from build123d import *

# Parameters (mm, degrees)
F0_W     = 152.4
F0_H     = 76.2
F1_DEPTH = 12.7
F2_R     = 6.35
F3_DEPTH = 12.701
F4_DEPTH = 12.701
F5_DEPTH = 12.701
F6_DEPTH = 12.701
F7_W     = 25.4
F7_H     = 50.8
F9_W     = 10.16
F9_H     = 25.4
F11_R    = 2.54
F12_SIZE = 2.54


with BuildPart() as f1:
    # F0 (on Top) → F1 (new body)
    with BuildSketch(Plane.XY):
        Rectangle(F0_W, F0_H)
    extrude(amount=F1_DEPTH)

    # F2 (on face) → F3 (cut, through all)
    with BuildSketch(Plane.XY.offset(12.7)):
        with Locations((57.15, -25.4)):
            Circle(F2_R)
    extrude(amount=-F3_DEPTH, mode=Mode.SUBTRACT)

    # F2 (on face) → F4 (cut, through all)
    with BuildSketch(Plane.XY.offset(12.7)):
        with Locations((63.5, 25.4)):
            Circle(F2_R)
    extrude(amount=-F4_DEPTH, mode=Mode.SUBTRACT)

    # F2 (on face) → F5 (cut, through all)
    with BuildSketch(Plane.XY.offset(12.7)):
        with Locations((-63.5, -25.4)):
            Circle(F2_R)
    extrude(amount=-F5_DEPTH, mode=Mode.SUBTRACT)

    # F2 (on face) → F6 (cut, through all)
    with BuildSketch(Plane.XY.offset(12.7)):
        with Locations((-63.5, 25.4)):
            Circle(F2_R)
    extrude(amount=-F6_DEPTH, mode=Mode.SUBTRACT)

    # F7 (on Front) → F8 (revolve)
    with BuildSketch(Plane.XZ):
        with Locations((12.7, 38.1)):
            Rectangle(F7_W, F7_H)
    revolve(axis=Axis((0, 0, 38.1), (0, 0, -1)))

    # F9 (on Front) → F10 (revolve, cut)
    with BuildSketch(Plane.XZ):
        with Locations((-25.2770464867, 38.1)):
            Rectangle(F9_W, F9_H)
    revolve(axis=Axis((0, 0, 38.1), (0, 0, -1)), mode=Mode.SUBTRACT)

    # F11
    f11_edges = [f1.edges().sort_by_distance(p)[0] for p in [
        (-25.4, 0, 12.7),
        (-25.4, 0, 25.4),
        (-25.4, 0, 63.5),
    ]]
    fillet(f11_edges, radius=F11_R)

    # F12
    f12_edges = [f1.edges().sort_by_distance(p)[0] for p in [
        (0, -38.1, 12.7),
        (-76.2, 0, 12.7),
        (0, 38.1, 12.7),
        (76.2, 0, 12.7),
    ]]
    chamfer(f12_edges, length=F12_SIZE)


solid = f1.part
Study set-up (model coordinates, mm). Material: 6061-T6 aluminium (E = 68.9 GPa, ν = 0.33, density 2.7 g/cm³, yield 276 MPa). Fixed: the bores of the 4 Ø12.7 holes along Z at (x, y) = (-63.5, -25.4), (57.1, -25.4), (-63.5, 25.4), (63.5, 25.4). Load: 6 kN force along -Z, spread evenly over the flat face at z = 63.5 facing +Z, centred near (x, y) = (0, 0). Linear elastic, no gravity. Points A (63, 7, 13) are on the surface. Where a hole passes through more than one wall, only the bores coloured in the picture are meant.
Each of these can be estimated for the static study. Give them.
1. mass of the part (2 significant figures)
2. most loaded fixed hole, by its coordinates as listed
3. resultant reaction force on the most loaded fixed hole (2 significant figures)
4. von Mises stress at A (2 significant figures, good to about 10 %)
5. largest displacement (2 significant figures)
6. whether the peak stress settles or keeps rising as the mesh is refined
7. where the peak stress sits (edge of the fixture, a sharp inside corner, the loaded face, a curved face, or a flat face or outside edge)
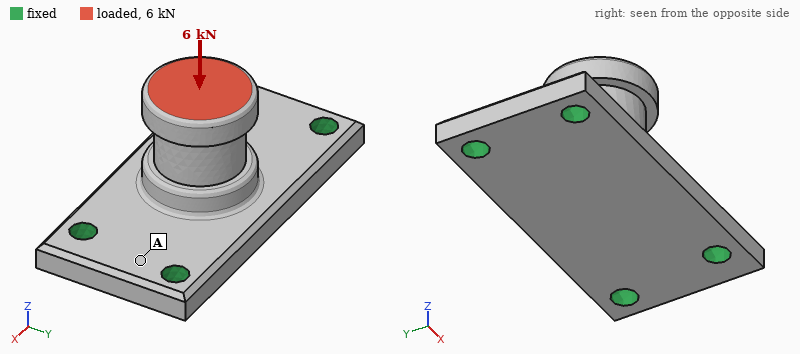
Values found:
600 g
(57.1, -25.4)
1.9 kN
8.0 MPa
39 µm
keeps rising
edge of the fixture
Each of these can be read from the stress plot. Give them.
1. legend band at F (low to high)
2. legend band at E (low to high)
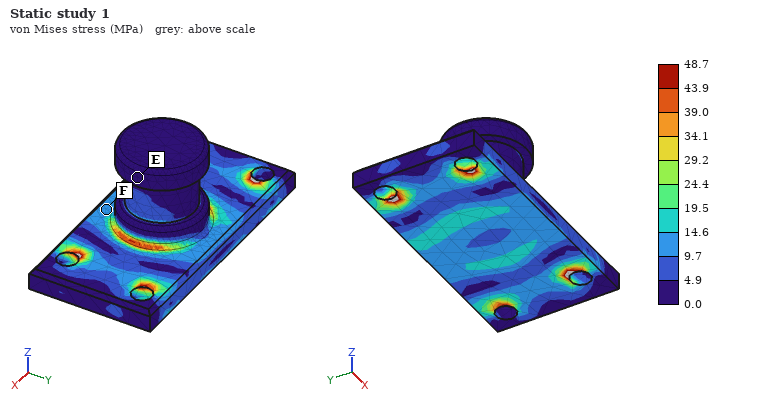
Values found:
9.7 to 14.6 MPa
0.0 to 4.9 MPa
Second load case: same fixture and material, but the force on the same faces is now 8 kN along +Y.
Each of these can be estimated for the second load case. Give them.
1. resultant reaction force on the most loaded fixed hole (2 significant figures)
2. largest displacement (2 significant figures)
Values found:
5.7 kN
0.29 mm
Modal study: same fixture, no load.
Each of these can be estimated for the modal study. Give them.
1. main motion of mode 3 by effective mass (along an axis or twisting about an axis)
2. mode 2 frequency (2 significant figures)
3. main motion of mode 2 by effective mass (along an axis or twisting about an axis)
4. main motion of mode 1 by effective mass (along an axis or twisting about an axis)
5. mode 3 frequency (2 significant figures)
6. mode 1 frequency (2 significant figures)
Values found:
along X
3400 Hz
along Z
along Y
4300 Hz
2700 Hz
